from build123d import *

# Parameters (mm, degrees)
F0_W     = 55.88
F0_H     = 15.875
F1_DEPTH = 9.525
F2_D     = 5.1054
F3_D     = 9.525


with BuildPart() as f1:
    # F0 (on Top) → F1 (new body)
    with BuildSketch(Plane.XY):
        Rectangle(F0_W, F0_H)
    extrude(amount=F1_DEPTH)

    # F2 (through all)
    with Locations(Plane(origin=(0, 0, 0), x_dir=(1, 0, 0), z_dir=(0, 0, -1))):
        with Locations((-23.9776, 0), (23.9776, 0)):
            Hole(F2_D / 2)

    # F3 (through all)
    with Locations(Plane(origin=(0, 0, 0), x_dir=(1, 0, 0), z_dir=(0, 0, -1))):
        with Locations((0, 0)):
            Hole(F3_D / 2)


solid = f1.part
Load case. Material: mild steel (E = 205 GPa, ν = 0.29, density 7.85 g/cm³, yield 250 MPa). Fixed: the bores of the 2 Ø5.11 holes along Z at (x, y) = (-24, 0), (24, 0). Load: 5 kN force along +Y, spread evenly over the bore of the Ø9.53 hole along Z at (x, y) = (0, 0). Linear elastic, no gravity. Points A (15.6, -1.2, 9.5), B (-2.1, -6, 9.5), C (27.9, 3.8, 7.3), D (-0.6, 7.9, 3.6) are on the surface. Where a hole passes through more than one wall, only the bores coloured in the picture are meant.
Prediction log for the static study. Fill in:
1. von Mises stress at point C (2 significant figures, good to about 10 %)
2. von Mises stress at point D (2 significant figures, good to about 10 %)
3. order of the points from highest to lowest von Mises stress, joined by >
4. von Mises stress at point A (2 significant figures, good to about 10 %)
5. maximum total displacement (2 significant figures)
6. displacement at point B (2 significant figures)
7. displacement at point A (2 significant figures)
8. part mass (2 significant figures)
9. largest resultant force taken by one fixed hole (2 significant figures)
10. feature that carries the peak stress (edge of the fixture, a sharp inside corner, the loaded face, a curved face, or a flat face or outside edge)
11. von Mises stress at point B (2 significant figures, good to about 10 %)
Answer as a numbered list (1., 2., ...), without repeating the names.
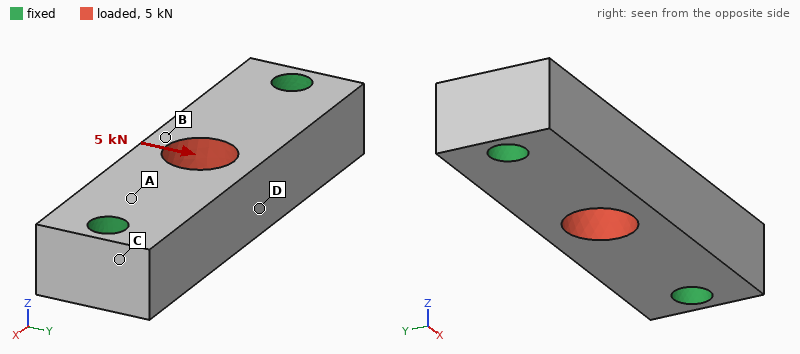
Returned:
1. 30 MPa
2. 100 MPa
3. D > B > A > C
4. 43 MPa
5. 13 µm
6. 12 µm
7. 4.5 µm
8. 58 g
9. 2.5 kN
10. edge of the fixture
11. 66 MPa
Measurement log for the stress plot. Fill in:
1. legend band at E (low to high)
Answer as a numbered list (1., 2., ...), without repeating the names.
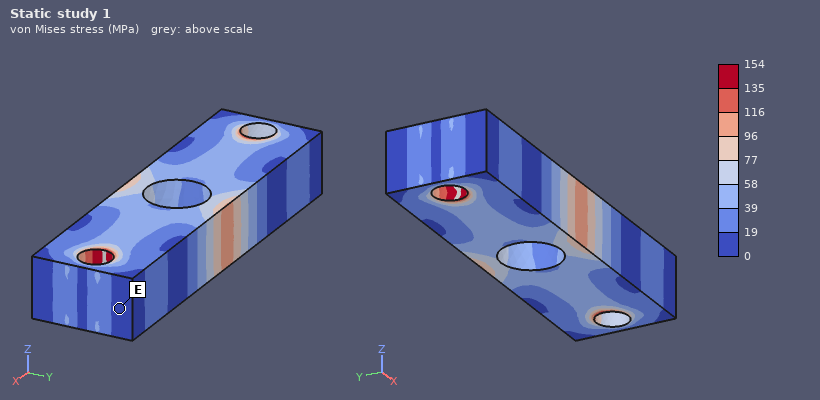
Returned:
1. 0 to 19 MPa
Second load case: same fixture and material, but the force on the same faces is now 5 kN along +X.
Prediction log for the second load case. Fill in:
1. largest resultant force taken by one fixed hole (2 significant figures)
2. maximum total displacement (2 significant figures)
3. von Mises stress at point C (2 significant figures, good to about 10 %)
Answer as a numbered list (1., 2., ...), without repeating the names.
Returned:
1. 2.5 kN
2. 2.1 µm
3. 6.5 MPa
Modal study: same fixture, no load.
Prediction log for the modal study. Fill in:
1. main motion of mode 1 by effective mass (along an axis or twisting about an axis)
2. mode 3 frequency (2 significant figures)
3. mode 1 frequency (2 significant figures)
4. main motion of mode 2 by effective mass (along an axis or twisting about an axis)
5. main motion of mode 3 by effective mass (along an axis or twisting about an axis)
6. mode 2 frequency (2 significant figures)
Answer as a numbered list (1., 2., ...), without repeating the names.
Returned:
1. along Z
2. 29 kHz
3. 19 kHz
4. along Y
5. twisting about X
6. 22 kHz
